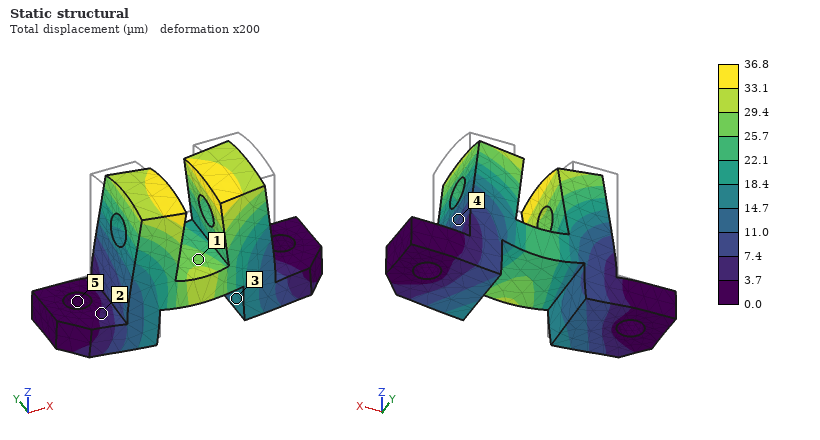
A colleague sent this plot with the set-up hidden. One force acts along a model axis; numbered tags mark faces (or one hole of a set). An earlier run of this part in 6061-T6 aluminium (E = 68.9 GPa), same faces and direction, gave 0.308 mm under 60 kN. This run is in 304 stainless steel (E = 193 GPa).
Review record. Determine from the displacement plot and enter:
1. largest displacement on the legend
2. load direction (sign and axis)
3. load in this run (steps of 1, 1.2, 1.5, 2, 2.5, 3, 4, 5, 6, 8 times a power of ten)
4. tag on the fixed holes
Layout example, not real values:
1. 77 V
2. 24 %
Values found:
1. 36.8 µm
2. -Z
3. 20 kN
4. 5
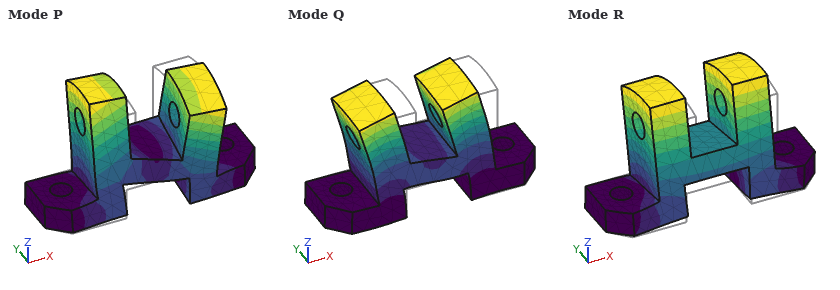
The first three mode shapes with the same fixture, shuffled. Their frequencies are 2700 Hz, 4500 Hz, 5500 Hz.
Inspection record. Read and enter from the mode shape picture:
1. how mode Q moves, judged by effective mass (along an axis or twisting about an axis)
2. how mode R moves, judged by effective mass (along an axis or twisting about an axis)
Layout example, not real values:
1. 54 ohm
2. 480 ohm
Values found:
1. along X
2. along Y
